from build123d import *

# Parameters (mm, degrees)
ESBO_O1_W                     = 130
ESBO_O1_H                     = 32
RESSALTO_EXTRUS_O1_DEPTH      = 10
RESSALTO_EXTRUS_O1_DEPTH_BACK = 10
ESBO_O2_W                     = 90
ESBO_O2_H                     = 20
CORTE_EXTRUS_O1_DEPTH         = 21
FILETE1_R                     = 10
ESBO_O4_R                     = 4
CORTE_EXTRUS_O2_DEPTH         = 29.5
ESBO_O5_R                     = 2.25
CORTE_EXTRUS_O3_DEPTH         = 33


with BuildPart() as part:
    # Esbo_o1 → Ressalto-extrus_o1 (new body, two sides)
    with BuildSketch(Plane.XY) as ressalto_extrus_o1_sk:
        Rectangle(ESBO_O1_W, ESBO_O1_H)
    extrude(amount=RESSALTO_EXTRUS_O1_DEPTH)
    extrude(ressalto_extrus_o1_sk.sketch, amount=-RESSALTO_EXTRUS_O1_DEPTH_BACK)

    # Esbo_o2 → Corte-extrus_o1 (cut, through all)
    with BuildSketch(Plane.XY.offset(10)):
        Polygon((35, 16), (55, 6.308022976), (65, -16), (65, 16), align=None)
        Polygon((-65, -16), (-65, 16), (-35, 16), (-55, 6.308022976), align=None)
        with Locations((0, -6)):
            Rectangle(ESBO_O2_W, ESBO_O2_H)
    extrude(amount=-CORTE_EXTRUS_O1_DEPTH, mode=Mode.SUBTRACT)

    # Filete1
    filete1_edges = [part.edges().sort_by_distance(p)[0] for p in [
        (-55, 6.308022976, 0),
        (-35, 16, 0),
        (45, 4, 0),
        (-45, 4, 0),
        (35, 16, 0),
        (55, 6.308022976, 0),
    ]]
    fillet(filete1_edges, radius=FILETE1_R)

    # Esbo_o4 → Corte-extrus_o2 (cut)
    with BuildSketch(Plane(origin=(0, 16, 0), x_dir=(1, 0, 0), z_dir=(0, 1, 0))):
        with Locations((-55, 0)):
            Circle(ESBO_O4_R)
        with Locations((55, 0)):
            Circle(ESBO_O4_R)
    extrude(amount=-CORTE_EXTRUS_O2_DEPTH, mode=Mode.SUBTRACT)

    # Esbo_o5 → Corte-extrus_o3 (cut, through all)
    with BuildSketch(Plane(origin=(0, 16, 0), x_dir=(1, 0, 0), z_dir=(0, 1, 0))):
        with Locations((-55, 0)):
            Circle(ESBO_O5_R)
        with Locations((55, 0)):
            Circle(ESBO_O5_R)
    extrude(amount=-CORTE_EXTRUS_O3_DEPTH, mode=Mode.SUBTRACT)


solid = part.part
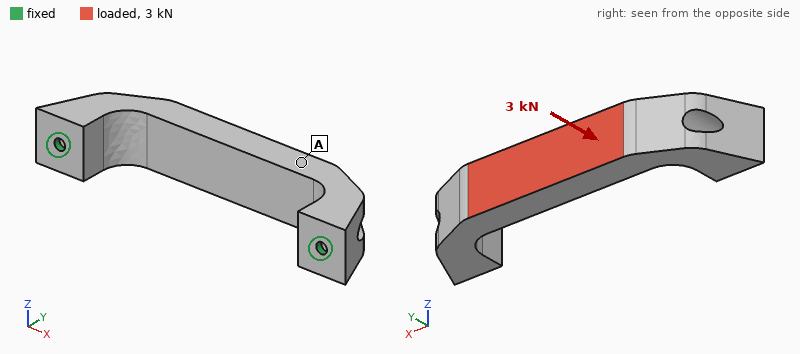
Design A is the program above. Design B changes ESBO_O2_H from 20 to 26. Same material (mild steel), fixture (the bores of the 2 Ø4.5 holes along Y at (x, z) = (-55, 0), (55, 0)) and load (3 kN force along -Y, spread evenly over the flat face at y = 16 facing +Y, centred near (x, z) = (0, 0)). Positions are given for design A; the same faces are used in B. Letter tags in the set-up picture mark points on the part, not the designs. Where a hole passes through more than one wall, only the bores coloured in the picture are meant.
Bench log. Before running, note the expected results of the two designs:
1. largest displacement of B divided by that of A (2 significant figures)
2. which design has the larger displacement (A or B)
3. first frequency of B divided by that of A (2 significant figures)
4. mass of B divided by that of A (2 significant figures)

1.9
B
1.1
0.84
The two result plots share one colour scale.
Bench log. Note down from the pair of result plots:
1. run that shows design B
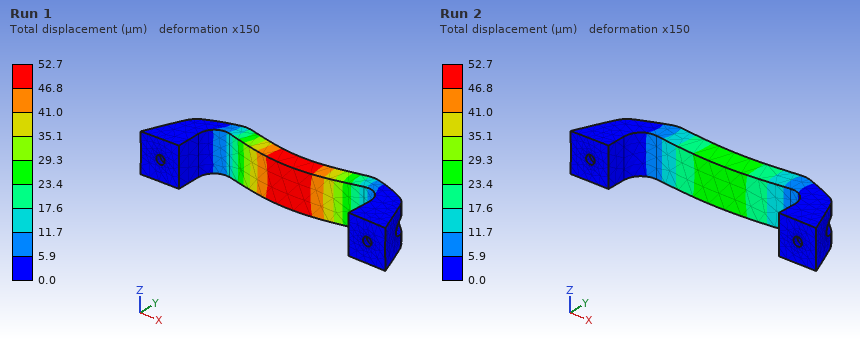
Run 1
